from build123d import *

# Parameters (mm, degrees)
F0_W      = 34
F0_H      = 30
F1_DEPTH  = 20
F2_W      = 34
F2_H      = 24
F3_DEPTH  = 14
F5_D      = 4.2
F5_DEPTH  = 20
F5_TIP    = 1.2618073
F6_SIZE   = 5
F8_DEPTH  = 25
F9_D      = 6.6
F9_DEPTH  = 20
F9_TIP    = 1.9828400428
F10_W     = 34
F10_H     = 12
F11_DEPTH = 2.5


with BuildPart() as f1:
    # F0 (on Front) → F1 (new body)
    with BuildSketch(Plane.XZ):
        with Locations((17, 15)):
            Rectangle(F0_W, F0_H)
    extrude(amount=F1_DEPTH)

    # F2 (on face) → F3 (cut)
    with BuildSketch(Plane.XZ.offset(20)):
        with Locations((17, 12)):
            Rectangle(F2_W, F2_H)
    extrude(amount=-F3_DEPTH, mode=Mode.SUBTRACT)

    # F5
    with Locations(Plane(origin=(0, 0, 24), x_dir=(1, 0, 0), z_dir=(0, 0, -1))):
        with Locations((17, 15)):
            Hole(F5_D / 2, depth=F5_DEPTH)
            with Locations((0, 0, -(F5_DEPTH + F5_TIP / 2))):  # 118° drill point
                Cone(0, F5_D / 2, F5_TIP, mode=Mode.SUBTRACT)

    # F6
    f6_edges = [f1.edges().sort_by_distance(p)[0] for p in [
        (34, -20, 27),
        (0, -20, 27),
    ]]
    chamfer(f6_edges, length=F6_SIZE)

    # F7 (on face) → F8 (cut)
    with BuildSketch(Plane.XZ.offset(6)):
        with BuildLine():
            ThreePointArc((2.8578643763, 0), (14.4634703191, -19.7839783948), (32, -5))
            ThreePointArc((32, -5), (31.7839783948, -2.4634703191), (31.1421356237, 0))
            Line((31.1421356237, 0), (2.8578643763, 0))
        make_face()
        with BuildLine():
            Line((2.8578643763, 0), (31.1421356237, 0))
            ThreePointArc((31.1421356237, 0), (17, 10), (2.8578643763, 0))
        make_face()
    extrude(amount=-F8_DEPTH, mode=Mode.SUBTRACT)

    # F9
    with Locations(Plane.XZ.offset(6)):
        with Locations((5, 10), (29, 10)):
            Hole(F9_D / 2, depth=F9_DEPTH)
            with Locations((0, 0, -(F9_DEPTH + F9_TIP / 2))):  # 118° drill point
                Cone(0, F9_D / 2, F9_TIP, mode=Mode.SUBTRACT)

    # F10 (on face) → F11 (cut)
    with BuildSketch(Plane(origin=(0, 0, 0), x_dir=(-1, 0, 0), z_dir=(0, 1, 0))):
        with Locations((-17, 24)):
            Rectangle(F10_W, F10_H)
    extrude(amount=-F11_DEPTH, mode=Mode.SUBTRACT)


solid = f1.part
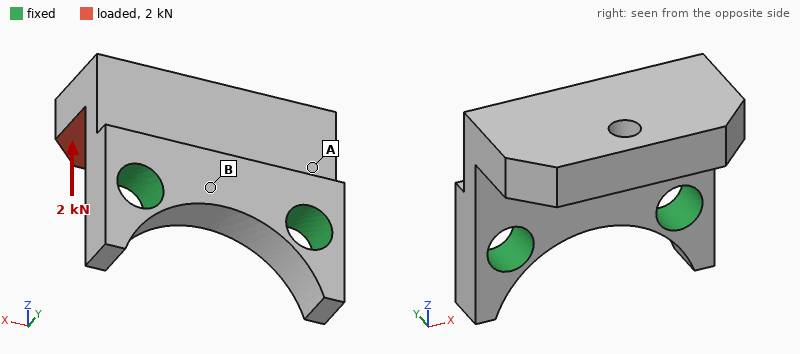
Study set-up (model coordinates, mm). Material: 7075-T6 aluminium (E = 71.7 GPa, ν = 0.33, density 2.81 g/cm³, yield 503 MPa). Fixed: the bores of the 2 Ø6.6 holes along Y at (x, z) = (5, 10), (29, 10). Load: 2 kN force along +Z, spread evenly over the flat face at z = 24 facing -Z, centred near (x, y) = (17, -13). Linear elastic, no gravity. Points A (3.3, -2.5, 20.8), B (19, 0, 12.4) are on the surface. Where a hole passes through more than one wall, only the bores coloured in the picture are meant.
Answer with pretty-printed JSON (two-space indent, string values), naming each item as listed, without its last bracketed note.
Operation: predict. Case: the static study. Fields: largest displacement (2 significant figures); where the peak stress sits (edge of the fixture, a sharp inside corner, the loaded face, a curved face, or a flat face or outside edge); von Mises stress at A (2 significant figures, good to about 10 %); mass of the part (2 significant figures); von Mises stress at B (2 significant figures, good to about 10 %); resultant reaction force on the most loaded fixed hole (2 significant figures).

{
  "largest displacement": "0.37 mm",
  "where the peak stress sits": "a flat face or outside edge",
  "von Mises stress at A": "210 MPa",
  "mass of the part": "17 g",
  "von Mises stress at B": "31 MPa",
  "resultant reaction force on the most loaded fixed hole": "1.1 kN"
}
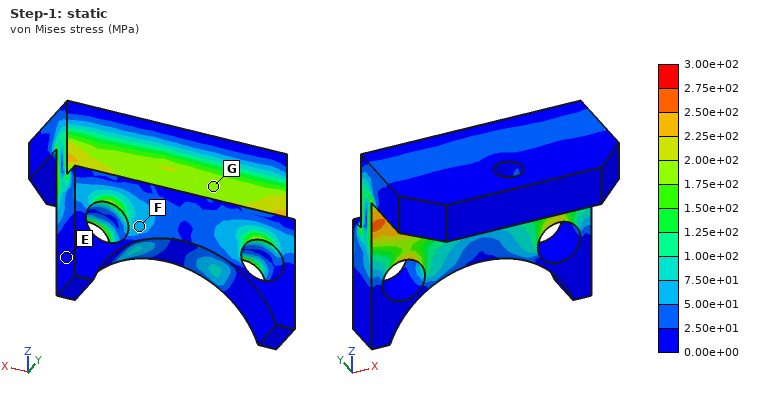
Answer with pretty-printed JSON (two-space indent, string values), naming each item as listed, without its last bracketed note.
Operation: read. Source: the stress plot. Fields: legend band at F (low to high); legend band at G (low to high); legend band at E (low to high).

{
  "legend band at F": "5.00e+01 to 7.50e+01 MPa",
  "legend band at G": "1.75e+02 to 2.00e+02 MPa",
  "legend band at E": "0.00e+00 to 2.50e+01 MPa"
}
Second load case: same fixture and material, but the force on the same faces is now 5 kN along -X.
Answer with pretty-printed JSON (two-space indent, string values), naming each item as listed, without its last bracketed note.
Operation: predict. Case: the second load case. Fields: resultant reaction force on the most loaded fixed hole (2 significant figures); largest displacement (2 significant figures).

{
  "resultant reaction force on the most loaded fixed hole": "3.8 kN",
  "largest displacement": "0.19 mm"
}
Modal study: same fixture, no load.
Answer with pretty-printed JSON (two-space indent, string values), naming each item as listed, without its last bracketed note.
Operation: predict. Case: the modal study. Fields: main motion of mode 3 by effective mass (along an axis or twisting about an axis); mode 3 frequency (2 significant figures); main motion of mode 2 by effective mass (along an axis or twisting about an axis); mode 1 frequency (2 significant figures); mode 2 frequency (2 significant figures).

{
  "main motion of mode 3 by effective mass": "along Y",
  "mode 3 frequency": "15 kHz",
  "main motion of mode 2 by effective mass": "along X",
  "mode 1 frequency": "4400 Hz",
  "mode 2 frequency": "9300 Hz"
}
